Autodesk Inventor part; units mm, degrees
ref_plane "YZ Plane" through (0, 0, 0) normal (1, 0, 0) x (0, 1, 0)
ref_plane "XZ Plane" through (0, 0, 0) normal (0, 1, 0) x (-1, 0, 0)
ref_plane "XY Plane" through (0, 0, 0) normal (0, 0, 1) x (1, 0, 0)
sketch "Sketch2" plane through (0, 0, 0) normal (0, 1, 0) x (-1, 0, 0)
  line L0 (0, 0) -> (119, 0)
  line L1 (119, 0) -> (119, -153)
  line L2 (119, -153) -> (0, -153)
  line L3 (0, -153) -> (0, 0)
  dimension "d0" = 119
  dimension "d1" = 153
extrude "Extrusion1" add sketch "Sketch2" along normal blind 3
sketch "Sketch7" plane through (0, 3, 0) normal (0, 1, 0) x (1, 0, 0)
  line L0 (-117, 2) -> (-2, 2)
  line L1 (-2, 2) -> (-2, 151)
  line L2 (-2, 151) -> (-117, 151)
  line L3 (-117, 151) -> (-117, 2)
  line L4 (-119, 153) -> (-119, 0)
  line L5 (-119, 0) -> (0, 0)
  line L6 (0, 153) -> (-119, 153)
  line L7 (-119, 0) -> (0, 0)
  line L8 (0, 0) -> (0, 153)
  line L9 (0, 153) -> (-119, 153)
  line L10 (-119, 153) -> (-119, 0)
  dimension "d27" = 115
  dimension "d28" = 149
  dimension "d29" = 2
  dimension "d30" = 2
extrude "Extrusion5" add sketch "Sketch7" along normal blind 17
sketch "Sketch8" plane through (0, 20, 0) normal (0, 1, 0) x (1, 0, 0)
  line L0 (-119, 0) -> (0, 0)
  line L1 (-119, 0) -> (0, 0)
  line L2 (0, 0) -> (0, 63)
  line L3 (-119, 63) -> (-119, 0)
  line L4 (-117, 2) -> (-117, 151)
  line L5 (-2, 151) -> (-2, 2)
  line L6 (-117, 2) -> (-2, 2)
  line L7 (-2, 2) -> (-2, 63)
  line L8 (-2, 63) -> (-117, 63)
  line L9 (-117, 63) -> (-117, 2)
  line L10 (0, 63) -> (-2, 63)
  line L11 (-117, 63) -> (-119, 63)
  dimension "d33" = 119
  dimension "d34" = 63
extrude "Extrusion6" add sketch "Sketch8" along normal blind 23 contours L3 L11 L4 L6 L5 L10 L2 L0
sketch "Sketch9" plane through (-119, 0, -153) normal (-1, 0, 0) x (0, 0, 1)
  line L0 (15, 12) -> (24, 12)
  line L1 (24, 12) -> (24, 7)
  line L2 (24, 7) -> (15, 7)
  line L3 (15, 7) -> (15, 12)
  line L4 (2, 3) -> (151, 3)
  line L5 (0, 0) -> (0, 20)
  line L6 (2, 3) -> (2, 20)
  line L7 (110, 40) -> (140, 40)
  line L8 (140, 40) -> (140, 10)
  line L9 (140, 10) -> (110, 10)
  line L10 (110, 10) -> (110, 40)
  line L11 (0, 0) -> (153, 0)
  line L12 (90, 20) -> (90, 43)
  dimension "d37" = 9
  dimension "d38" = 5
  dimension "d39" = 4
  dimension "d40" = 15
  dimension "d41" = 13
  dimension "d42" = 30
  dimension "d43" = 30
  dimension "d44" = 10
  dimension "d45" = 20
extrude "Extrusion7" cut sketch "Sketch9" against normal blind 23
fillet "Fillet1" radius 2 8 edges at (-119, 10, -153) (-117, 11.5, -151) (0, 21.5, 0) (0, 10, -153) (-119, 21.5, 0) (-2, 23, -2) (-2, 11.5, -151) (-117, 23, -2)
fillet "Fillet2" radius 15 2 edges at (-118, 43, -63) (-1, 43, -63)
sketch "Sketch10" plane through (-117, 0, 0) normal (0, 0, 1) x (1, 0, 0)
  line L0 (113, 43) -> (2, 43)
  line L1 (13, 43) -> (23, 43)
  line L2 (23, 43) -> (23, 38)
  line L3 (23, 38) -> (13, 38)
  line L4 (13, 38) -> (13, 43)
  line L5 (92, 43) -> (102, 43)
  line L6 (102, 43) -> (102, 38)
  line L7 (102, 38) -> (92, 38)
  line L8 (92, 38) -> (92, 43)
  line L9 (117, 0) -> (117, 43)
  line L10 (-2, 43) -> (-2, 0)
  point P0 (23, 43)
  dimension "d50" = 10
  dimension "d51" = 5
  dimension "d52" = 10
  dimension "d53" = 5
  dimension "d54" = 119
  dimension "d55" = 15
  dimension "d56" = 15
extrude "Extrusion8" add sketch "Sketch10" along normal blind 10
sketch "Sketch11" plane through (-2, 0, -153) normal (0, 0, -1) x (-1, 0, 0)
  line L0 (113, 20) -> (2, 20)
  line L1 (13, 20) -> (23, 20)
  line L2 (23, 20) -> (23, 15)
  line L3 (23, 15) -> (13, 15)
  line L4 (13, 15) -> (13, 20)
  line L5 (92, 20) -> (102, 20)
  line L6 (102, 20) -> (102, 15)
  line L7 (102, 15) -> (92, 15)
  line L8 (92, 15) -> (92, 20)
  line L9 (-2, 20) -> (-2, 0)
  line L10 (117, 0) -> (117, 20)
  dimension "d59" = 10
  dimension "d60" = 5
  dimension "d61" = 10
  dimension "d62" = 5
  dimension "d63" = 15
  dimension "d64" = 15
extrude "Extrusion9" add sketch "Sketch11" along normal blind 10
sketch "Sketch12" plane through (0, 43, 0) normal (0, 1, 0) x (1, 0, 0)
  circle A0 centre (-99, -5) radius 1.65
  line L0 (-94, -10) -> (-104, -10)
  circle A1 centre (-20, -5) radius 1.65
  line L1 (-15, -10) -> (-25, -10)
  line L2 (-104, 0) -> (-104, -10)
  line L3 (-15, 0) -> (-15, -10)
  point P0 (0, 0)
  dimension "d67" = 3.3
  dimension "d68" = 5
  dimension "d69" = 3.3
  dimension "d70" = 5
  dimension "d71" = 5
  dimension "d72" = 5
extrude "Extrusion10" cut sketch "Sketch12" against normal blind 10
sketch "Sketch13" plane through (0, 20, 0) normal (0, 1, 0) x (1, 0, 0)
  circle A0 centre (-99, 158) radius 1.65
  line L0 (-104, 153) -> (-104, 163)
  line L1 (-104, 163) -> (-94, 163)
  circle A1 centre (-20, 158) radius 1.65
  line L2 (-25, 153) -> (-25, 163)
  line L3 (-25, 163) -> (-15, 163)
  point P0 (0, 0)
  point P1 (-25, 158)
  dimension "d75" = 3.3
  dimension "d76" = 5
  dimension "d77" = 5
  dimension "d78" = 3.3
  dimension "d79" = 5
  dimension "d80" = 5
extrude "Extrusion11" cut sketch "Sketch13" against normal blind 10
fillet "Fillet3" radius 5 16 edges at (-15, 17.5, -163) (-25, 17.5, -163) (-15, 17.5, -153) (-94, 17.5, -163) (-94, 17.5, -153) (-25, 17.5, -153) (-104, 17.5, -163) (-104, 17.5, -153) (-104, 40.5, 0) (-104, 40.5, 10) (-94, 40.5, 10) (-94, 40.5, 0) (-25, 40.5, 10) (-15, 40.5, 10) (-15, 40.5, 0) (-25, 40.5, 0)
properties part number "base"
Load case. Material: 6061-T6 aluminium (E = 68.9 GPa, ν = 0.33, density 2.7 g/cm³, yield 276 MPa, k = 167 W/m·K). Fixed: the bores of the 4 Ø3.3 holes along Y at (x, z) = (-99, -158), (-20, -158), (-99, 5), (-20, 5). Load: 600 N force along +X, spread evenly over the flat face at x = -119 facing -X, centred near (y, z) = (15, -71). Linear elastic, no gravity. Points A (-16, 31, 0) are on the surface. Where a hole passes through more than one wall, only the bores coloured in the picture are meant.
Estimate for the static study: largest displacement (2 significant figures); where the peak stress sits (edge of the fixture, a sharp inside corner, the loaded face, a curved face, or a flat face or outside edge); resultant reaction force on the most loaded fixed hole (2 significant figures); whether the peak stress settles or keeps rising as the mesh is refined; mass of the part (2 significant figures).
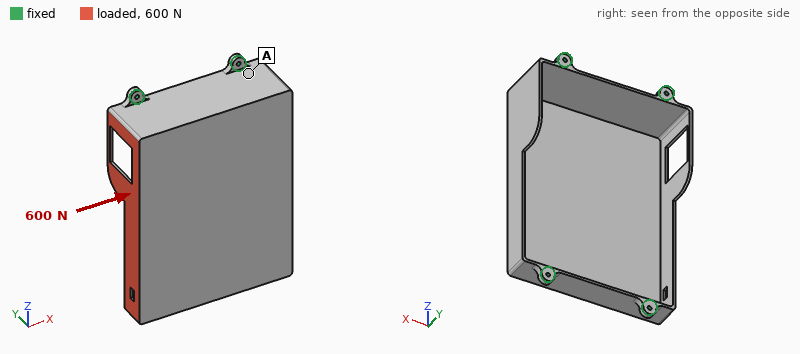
0.74 mm
a sharp inside corner
220 N
keeps rising
230 g
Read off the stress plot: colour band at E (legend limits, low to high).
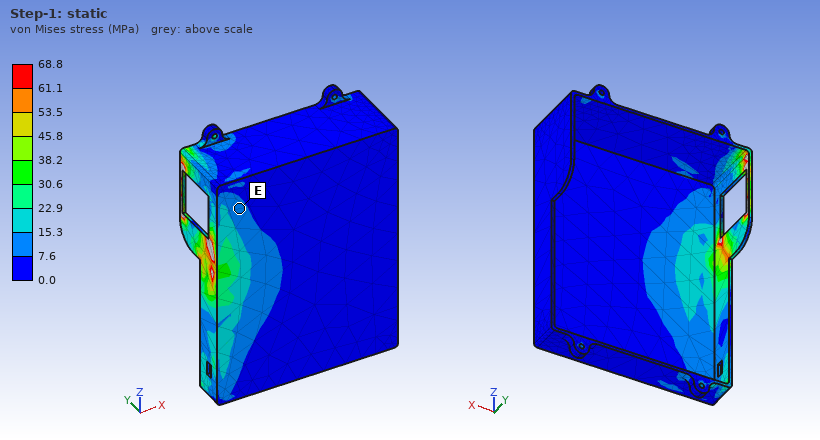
7.6 to 15.3 MPa
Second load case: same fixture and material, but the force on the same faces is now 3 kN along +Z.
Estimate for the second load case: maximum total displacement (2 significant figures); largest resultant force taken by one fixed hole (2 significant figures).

0.45 mm
1.3 kN
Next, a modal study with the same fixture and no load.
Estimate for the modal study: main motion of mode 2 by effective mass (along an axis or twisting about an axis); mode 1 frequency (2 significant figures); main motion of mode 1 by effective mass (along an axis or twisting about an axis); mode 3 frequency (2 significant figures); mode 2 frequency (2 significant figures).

along Z
850 Hz
along Y
1500 Hz
1300 Hz
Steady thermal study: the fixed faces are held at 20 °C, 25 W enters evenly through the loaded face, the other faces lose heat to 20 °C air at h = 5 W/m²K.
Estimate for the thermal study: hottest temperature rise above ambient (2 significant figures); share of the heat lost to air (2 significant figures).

38 K
16 %
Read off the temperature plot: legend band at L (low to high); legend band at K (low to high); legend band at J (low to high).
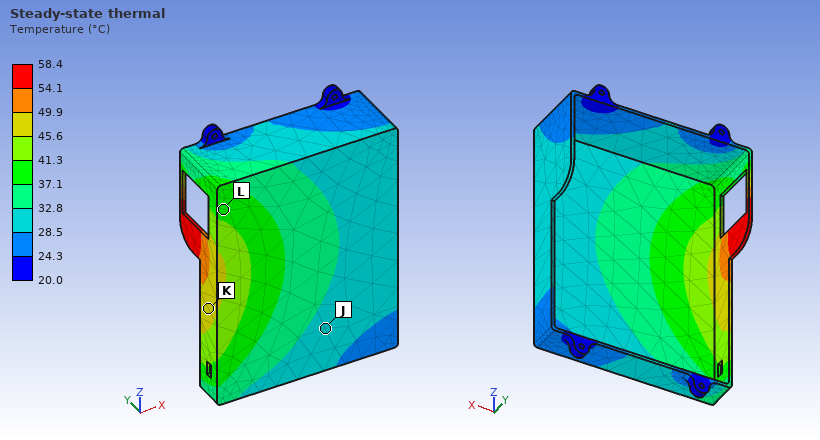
37.1 to 41.3 °C
45.6 to 49.9 °C
28.5 to 32.8 °C
